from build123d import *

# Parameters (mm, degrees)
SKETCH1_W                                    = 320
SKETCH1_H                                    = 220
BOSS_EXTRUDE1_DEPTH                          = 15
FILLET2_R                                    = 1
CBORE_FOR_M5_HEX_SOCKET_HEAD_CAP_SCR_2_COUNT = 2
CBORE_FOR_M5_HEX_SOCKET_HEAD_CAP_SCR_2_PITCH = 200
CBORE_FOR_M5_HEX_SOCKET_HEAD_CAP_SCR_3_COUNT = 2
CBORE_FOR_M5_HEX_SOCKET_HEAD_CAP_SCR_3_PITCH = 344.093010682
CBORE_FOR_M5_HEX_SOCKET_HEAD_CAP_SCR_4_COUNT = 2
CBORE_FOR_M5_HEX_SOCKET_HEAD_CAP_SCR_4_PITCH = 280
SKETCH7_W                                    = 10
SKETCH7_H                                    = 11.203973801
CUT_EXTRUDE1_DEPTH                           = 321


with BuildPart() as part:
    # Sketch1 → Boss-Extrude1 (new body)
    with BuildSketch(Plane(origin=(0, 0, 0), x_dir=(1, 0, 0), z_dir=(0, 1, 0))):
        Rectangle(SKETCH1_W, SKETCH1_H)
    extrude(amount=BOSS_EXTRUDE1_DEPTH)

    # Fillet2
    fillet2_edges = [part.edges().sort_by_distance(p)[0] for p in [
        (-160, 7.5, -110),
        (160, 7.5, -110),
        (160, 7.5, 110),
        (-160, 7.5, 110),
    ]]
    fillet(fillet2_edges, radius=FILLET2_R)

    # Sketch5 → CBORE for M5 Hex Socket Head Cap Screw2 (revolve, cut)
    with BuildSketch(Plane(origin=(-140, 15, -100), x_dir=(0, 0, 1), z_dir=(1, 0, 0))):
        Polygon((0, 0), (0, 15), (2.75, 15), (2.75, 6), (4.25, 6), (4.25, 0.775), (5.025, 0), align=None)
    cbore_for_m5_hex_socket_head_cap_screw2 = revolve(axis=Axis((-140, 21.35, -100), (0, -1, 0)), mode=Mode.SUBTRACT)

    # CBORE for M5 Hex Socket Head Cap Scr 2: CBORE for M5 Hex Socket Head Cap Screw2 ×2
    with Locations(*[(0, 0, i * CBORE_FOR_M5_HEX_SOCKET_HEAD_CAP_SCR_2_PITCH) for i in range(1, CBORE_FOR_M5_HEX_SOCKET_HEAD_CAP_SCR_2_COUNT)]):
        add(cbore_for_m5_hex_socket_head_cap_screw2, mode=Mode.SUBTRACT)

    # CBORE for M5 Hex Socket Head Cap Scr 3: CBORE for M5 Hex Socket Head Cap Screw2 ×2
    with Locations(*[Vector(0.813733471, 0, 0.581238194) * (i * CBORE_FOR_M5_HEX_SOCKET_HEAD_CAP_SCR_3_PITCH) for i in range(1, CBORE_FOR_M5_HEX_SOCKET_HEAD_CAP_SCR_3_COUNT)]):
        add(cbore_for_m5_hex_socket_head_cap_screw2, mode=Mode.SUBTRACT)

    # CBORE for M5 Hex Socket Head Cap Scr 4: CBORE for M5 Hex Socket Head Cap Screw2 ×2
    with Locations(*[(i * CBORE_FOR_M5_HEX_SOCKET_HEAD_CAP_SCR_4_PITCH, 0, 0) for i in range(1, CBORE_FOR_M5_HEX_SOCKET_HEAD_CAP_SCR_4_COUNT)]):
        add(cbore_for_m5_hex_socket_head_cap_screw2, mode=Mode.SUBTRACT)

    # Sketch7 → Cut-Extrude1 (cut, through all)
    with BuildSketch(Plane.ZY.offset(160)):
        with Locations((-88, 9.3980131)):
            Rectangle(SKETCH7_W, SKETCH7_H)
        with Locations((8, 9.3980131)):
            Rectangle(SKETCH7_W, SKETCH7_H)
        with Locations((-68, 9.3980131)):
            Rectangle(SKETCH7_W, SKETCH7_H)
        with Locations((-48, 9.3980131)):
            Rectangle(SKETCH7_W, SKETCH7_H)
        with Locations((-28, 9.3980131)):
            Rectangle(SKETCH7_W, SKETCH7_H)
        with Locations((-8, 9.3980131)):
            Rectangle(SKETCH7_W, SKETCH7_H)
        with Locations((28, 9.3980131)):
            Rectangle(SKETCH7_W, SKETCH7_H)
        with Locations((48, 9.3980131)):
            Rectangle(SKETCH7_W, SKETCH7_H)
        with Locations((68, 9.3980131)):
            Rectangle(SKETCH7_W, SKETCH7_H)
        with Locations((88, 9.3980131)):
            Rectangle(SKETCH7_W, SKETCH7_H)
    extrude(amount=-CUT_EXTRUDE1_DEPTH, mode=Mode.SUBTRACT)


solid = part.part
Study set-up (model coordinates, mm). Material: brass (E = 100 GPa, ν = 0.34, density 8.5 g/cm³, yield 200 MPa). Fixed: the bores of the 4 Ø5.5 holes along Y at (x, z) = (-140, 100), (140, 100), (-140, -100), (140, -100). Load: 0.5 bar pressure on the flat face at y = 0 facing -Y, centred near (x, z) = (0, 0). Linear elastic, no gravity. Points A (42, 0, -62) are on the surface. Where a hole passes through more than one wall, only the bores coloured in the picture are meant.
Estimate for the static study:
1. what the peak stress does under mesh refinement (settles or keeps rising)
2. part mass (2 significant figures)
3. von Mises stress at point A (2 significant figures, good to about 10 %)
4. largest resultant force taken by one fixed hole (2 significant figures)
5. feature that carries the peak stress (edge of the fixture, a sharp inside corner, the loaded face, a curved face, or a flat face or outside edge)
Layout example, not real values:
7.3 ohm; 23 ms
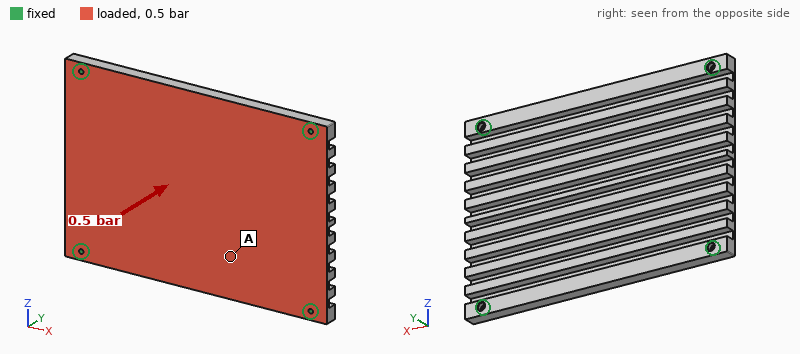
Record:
keeps rising; 5.9 kg; 8.3 MPa; 1000 N; edge of the fixture
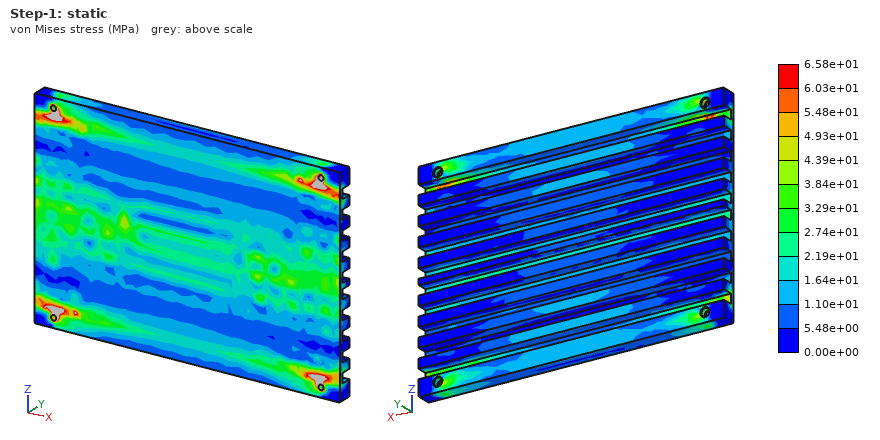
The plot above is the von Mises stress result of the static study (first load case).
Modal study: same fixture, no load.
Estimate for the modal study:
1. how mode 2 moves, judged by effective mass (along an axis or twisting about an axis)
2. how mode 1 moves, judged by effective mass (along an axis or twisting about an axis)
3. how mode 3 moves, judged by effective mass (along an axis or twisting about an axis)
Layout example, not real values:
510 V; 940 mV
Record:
twisting about Z; along Y; twisting about X
